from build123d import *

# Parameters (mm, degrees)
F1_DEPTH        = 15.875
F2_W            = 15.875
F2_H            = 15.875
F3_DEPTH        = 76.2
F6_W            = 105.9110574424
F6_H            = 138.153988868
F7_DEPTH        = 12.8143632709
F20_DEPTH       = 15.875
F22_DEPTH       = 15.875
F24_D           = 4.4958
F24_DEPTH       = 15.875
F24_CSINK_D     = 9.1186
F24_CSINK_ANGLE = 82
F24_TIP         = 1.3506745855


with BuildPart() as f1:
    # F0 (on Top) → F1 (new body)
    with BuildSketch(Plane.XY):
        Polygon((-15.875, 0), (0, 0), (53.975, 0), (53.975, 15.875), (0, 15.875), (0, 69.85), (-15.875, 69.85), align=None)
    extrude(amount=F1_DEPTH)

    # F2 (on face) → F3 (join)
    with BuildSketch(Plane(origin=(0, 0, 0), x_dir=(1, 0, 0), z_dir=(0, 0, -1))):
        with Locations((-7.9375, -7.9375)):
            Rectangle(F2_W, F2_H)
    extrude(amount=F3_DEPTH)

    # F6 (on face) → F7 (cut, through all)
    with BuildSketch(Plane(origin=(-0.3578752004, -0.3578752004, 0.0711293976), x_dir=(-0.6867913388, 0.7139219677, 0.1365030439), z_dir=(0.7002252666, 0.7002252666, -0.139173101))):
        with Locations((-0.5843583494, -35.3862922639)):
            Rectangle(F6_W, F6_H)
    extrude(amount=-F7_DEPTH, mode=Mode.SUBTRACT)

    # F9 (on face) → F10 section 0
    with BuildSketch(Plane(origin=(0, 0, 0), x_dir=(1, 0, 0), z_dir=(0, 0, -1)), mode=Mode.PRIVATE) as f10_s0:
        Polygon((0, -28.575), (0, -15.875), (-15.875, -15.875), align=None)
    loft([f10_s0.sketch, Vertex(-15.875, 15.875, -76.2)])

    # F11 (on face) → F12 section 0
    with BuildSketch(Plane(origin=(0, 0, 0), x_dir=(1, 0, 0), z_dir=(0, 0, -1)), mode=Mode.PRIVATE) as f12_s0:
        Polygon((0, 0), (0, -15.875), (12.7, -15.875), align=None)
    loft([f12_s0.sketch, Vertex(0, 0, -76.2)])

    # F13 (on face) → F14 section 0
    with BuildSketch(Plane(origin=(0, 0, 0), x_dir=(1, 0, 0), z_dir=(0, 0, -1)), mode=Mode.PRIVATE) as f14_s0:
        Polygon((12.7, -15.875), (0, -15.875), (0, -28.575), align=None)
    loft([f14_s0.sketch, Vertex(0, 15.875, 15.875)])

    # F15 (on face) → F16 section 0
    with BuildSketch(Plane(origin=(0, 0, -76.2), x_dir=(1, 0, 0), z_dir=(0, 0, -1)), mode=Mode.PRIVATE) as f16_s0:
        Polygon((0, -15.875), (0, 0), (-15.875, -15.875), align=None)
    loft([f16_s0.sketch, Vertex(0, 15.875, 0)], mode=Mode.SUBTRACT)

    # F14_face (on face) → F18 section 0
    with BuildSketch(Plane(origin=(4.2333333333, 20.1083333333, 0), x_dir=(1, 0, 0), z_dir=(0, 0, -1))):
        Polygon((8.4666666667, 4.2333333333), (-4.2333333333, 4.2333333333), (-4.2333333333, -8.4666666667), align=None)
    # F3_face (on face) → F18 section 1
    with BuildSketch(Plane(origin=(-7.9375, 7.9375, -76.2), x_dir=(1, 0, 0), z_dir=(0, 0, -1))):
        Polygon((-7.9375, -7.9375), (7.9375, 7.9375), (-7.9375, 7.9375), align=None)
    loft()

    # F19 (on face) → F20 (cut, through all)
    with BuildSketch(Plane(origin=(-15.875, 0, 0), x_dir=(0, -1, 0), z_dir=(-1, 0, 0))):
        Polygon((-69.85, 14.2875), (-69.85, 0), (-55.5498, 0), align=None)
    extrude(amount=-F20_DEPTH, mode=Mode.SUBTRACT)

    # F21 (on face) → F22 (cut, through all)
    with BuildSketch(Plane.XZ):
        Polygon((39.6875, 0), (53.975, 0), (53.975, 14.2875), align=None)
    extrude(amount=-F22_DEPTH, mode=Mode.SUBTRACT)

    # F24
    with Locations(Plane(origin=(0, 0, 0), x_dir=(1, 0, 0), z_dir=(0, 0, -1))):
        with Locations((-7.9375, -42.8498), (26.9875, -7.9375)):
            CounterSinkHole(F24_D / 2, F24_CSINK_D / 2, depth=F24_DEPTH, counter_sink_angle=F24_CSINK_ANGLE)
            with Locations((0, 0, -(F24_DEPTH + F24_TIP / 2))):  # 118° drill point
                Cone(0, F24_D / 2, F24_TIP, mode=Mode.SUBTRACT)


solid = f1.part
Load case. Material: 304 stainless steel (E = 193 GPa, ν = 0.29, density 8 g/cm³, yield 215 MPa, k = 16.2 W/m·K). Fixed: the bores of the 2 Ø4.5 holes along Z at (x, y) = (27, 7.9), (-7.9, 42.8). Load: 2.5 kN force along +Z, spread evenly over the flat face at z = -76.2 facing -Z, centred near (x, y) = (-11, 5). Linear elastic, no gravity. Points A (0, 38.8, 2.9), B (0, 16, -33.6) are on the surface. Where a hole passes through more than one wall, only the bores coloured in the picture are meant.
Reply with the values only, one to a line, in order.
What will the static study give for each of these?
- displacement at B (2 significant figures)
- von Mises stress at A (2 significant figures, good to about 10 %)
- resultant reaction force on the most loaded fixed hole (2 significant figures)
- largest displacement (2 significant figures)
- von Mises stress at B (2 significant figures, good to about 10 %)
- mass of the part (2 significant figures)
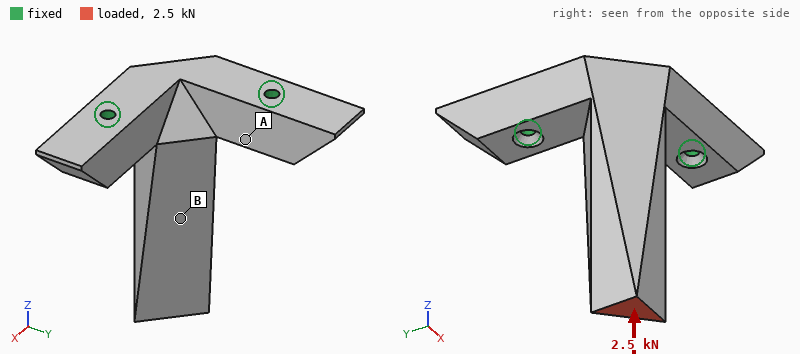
0.044 mm
29 MPa
1.3 kN
0.12 mm
14 MPa
390 g
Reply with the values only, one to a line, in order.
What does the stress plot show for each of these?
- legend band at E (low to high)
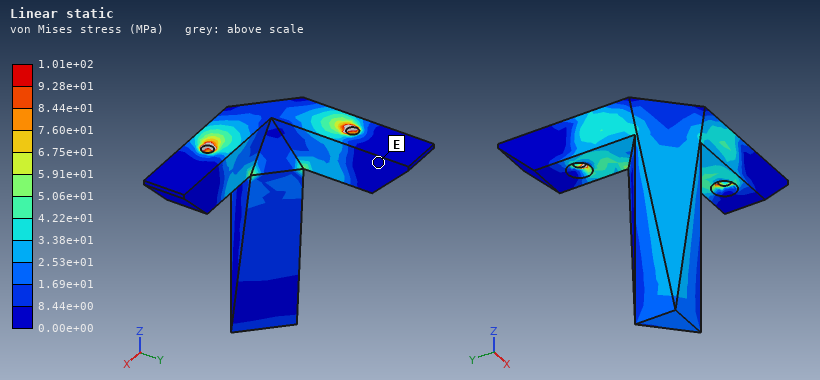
0.00e+00 to 8.44e+00 MPa
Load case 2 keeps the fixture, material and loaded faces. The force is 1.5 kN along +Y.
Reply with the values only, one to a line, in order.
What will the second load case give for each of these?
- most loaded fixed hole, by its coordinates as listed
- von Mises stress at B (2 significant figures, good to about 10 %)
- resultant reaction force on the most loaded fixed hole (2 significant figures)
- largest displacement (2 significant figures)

(-7.9, 42.8)
57 MPa
2.8 kN
0.27 mm
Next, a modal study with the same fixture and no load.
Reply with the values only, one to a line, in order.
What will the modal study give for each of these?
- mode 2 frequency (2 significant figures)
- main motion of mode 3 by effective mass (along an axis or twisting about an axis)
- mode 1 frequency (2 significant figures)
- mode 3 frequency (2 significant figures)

2600 Hz
along Z
1700 Hz
6900 Hz
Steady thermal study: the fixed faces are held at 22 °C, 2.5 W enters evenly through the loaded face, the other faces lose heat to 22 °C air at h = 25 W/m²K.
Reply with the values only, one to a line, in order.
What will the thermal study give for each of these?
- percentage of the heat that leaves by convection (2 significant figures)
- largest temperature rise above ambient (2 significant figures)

67 %
34 K
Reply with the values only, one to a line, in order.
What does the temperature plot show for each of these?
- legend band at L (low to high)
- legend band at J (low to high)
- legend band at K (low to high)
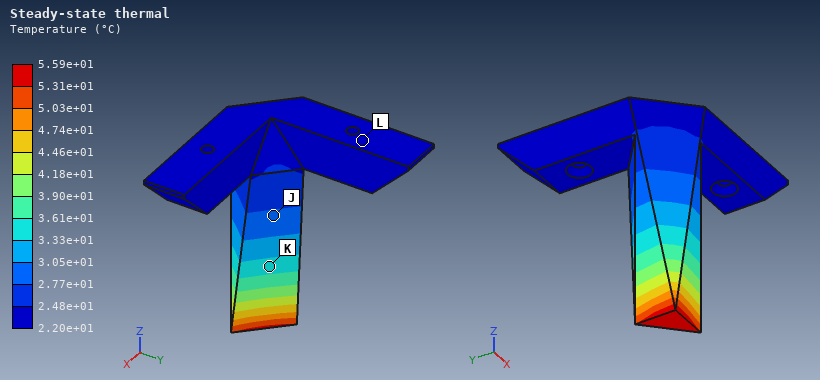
2.20e+01 to 2.48e+01 °C
2.77e+01 to 3.05e+01 °C
3.33e+01 to 3.61e+01 °C
